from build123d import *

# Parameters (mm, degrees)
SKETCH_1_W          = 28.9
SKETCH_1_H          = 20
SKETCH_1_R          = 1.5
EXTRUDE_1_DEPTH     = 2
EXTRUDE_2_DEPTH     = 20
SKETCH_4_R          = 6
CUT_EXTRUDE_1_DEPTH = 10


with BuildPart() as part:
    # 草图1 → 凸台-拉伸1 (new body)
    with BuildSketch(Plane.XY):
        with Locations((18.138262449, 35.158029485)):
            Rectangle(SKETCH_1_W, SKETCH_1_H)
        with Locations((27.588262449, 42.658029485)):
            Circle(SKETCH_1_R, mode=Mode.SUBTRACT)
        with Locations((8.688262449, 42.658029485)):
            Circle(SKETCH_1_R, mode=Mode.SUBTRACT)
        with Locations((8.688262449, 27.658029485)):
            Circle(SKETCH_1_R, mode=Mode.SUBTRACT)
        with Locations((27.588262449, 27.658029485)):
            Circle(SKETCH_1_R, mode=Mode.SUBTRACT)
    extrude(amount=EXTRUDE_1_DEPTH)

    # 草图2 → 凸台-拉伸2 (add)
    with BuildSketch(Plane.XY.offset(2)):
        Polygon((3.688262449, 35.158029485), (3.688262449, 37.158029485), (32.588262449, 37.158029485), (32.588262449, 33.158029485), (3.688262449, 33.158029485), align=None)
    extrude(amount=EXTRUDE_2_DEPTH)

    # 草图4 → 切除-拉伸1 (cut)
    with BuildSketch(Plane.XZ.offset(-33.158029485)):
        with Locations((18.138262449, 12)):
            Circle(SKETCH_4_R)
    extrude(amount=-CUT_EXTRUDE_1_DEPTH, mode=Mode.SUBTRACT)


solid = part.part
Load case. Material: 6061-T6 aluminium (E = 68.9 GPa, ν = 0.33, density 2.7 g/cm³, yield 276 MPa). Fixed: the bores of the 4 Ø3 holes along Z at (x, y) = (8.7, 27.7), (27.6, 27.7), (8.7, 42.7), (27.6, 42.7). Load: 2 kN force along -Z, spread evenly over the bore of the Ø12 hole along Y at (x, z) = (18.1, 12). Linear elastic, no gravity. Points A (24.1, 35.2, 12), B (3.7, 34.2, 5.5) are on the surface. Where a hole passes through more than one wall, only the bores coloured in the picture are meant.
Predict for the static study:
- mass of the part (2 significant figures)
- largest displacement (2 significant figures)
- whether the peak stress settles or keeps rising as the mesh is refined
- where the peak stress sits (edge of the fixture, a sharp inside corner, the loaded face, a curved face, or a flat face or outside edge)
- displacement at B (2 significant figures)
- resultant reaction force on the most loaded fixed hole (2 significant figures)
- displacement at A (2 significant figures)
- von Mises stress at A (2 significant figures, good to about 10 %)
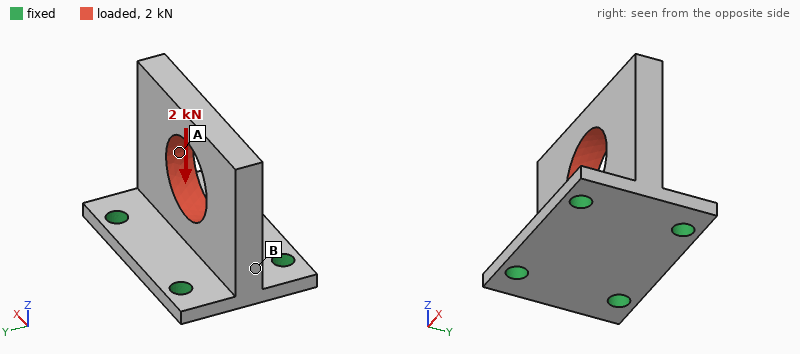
8.0 g
32 µm
keeps rising
edge of the fixture
22 µm
520 N
26 µm
52 MPa
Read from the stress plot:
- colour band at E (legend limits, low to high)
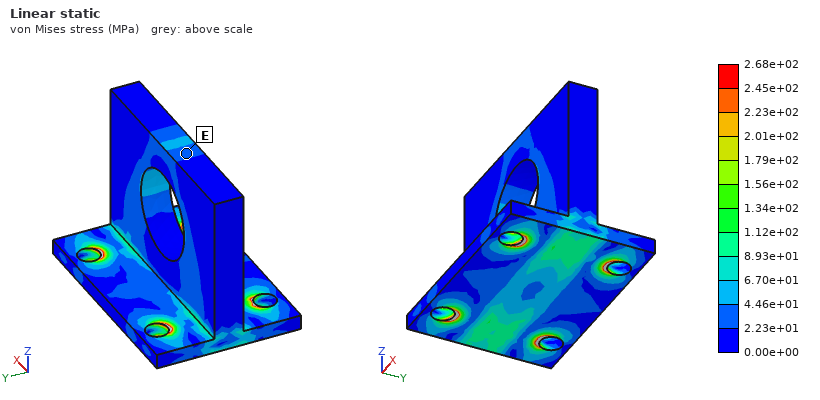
2.23e+01 to 4.46e+01 MPa
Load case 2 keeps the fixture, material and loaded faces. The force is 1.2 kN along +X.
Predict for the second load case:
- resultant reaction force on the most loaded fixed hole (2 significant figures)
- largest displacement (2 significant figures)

470 N
63 µm
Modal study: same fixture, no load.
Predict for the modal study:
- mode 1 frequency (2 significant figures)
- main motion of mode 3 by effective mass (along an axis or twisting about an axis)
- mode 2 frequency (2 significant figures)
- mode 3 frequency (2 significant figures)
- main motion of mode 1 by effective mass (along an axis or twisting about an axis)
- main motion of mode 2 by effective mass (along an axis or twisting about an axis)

5500 Hz
along X
10 kHz
11 kHz
along Y
twisting about Z
